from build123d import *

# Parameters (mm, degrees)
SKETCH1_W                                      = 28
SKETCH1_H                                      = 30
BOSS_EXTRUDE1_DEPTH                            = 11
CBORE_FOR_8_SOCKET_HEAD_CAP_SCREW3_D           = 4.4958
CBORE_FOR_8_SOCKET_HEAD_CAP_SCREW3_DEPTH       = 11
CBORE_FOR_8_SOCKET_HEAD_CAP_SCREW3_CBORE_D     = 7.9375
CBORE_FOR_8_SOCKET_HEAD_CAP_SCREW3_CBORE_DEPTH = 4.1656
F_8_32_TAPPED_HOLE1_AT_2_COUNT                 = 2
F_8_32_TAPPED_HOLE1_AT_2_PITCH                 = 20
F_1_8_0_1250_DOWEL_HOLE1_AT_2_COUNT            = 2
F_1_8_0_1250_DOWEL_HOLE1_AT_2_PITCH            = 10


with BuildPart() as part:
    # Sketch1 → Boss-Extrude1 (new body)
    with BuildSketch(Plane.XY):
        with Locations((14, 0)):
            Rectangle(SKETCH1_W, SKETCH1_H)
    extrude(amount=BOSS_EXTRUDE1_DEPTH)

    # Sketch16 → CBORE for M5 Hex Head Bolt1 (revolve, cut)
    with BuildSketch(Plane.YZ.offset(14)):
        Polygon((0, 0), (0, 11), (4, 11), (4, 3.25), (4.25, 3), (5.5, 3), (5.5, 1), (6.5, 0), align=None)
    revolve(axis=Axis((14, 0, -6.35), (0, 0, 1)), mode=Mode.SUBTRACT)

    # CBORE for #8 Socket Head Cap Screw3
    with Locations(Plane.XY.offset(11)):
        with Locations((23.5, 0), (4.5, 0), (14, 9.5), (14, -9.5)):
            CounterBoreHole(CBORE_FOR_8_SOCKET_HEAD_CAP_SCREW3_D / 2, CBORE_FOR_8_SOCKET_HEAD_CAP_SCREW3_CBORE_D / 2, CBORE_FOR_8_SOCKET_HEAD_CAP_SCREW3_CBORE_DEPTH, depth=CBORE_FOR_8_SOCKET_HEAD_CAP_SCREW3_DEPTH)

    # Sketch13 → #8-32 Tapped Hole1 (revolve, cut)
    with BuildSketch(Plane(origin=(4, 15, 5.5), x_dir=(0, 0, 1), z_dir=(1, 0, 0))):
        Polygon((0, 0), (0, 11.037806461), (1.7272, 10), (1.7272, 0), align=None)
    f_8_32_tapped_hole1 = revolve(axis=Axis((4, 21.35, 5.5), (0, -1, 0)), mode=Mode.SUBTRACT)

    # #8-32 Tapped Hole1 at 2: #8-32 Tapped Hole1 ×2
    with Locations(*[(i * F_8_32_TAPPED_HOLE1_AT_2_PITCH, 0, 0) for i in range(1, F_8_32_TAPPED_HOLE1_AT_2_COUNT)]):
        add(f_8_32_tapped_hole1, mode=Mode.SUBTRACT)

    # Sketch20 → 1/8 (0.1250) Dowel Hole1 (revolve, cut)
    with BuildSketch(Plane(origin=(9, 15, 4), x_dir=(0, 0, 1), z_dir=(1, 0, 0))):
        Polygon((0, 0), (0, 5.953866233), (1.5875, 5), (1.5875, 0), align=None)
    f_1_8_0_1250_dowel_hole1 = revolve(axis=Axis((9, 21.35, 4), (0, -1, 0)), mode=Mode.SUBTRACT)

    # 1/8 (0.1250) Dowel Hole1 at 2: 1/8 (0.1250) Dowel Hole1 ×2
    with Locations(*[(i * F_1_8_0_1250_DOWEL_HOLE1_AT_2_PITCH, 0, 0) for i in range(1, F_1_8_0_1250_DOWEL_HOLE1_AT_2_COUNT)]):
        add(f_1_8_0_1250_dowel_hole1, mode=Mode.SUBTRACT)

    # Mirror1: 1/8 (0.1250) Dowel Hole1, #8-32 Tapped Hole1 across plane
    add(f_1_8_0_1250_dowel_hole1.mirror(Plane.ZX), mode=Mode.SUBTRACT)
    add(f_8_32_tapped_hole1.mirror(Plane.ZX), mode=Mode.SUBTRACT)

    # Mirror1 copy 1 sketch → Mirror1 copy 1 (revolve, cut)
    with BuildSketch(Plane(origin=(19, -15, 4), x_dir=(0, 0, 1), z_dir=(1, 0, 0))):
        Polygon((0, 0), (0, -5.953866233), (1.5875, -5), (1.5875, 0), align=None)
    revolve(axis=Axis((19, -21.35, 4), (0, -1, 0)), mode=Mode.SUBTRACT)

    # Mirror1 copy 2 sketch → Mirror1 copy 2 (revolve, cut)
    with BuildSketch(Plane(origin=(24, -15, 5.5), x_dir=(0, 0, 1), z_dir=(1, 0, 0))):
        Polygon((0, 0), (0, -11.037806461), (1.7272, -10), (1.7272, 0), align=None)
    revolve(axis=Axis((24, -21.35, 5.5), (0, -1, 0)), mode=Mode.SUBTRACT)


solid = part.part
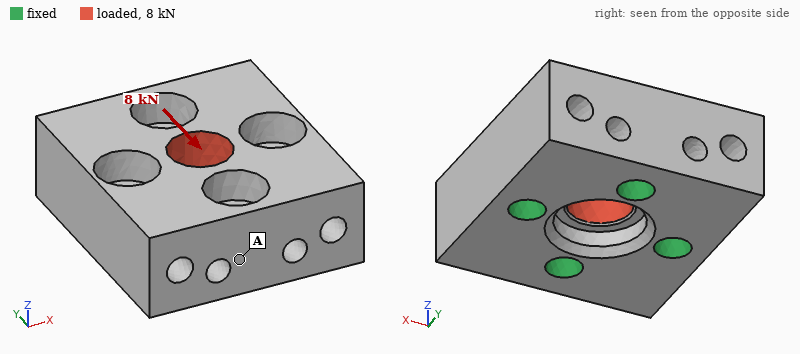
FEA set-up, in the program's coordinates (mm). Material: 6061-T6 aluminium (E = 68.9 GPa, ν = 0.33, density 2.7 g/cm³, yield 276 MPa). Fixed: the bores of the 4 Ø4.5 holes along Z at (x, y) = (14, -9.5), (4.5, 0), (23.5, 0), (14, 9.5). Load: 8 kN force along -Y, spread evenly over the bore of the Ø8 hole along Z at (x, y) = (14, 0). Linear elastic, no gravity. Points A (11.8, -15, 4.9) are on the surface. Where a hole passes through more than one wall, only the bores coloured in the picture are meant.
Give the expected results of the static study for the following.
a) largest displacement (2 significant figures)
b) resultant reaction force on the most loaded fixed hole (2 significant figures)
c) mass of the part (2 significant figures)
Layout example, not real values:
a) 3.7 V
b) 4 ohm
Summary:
a) 15 µm
b) 2.5 kN
c) 18 g
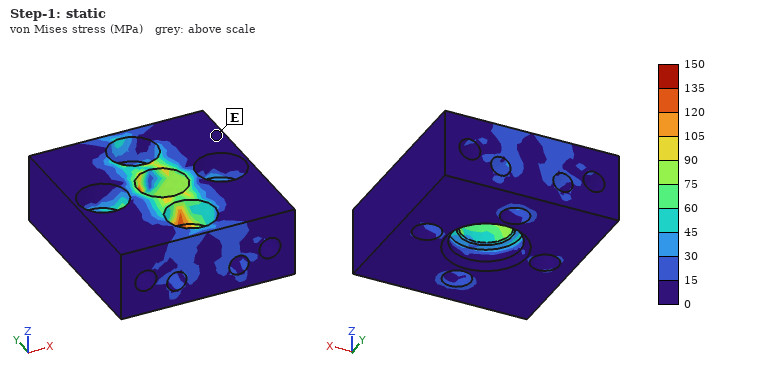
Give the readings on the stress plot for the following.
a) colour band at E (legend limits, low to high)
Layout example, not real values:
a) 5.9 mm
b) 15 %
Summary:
a) 0 to 15 MPa
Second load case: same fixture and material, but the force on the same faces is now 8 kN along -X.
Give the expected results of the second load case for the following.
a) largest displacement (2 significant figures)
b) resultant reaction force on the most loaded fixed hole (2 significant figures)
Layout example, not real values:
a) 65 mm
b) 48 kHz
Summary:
a) 15 µm
b) 2.5 kN
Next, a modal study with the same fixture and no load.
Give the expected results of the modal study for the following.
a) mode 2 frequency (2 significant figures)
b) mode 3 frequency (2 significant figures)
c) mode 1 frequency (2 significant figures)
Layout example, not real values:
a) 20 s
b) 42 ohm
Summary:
a) 37 kHz
b) 37 kHz
c) 35 kHz
